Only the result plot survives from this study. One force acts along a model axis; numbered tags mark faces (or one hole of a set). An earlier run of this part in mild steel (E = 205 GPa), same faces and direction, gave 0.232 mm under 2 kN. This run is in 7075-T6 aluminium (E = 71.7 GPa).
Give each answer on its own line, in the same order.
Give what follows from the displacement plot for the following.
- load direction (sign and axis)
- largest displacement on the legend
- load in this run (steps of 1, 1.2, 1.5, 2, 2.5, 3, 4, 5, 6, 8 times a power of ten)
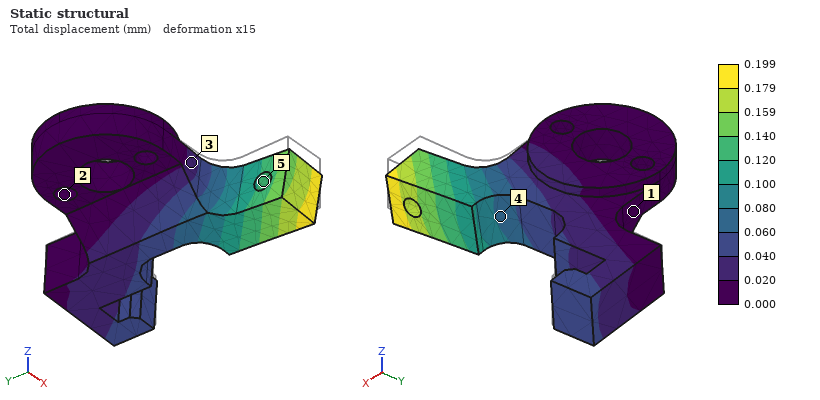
-Z
0.199 mm
600 N
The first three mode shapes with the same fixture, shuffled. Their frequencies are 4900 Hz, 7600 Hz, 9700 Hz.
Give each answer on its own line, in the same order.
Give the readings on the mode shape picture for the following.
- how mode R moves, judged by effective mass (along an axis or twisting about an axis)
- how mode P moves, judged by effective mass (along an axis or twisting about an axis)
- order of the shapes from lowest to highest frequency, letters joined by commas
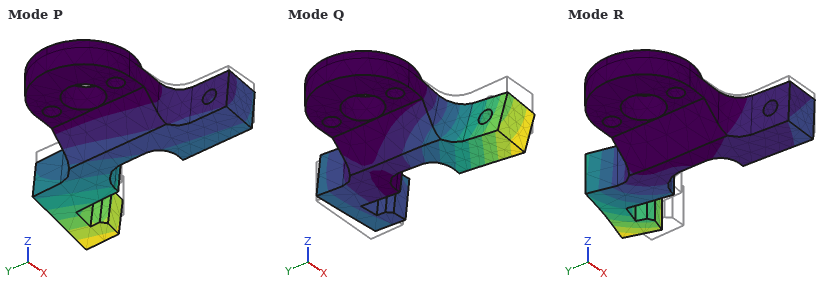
along Y
along Z
P, Q, R
